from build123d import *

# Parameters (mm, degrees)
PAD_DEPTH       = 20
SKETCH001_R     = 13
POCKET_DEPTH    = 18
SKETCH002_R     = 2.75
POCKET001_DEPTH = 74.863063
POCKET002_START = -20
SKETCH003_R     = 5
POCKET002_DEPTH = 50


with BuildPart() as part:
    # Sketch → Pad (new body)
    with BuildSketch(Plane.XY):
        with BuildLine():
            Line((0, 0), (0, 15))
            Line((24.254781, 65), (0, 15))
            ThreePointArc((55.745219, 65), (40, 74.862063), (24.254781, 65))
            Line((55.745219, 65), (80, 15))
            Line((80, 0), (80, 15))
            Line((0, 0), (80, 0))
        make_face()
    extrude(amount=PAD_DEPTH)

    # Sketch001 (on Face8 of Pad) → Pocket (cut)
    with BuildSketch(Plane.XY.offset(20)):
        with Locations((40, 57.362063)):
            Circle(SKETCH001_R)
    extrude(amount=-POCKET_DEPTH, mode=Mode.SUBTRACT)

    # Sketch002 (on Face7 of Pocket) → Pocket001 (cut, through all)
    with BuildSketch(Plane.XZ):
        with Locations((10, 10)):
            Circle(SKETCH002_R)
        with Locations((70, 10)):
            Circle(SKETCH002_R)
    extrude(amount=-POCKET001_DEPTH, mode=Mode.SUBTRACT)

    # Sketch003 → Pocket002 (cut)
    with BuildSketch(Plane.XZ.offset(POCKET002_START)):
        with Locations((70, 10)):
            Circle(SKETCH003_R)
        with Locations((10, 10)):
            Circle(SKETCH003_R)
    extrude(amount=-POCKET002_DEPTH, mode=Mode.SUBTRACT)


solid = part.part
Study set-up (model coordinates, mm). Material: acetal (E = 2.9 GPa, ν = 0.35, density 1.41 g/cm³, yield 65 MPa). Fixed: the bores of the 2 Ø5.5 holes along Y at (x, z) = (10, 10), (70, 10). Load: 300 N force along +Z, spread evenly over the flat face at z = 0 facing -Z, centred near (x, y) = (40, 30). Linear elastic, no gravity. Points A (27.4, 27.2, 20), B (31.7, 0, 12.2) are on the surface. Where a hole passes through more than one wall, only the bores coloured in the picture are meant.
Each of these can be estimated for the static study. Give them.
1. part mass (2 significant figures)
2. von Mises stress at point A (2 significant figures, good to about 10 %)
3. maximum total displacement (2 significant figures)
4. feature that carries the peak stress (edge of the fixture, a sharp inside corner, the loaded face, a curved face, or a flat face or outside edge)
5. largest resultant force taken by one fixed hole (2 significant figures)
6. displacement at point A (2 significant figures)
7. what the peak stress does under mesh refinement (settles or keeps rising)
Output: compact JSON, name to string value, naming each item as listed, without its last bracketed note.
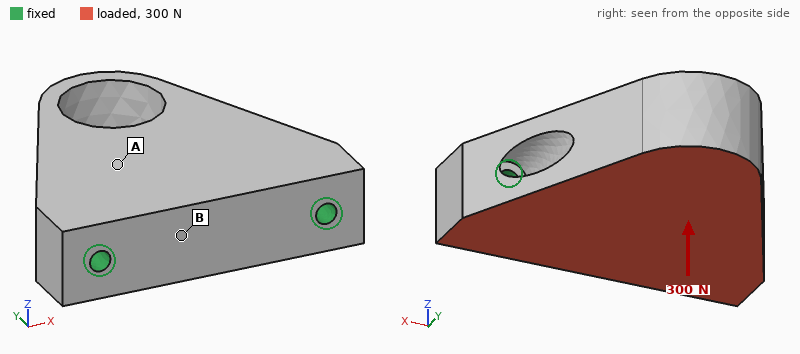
{"part mass": "100 g", "von Mises stress at point A": "0.79 MPa", "maximum total displacement": "0.11 mm", "feature that carries the peak stress": "edge of the fixture", "largest resultant force taken by one fixed hole": "150 N", "displacement at point A": "0.029 mm", "what the peak stress does under mesh refinement": "keeps rising"}
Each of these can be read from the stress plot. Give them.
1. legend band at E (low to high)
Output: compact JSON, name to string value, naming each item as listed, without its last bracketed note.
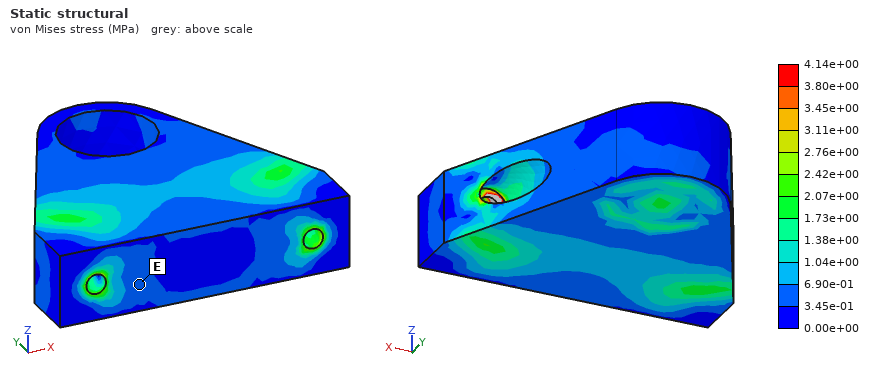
{"legend band at E": "3.45e-01 to 6.90e-01 MPa"}
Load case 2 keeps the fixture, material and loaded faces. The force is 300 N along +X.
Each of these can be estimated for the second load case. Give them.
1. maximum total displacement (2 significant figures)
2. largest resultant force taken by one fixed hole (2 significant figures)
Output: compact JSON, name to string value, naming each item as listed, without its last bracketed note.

{"maximum total displacement": "18 µm", "largest resultant force taken by one fixed hole": "180 N"}
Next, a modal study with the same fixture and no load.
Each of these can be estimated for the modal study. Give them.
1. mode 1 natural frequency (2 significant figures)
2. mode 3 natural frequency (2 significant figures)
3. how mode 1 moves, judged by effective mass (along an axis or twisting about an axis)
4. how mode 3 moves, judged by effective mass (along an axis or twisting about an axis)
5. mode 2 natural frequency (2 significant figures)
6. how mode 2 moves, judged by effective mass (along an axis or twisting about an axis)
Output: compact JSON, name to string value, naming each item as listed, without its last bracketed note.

{"mode 1 natural frequency": "1200 Hz", "mode 3 natural frequency": "3500 Hz", "how mode 1 moves, judged by effective mass": "along Z", "how mode 3 moves, judged by effective mass": "along X", "mode 2 natural frequency": "3100 Hz", "how mode 2 moves, judged by effective mass": "along X"}
